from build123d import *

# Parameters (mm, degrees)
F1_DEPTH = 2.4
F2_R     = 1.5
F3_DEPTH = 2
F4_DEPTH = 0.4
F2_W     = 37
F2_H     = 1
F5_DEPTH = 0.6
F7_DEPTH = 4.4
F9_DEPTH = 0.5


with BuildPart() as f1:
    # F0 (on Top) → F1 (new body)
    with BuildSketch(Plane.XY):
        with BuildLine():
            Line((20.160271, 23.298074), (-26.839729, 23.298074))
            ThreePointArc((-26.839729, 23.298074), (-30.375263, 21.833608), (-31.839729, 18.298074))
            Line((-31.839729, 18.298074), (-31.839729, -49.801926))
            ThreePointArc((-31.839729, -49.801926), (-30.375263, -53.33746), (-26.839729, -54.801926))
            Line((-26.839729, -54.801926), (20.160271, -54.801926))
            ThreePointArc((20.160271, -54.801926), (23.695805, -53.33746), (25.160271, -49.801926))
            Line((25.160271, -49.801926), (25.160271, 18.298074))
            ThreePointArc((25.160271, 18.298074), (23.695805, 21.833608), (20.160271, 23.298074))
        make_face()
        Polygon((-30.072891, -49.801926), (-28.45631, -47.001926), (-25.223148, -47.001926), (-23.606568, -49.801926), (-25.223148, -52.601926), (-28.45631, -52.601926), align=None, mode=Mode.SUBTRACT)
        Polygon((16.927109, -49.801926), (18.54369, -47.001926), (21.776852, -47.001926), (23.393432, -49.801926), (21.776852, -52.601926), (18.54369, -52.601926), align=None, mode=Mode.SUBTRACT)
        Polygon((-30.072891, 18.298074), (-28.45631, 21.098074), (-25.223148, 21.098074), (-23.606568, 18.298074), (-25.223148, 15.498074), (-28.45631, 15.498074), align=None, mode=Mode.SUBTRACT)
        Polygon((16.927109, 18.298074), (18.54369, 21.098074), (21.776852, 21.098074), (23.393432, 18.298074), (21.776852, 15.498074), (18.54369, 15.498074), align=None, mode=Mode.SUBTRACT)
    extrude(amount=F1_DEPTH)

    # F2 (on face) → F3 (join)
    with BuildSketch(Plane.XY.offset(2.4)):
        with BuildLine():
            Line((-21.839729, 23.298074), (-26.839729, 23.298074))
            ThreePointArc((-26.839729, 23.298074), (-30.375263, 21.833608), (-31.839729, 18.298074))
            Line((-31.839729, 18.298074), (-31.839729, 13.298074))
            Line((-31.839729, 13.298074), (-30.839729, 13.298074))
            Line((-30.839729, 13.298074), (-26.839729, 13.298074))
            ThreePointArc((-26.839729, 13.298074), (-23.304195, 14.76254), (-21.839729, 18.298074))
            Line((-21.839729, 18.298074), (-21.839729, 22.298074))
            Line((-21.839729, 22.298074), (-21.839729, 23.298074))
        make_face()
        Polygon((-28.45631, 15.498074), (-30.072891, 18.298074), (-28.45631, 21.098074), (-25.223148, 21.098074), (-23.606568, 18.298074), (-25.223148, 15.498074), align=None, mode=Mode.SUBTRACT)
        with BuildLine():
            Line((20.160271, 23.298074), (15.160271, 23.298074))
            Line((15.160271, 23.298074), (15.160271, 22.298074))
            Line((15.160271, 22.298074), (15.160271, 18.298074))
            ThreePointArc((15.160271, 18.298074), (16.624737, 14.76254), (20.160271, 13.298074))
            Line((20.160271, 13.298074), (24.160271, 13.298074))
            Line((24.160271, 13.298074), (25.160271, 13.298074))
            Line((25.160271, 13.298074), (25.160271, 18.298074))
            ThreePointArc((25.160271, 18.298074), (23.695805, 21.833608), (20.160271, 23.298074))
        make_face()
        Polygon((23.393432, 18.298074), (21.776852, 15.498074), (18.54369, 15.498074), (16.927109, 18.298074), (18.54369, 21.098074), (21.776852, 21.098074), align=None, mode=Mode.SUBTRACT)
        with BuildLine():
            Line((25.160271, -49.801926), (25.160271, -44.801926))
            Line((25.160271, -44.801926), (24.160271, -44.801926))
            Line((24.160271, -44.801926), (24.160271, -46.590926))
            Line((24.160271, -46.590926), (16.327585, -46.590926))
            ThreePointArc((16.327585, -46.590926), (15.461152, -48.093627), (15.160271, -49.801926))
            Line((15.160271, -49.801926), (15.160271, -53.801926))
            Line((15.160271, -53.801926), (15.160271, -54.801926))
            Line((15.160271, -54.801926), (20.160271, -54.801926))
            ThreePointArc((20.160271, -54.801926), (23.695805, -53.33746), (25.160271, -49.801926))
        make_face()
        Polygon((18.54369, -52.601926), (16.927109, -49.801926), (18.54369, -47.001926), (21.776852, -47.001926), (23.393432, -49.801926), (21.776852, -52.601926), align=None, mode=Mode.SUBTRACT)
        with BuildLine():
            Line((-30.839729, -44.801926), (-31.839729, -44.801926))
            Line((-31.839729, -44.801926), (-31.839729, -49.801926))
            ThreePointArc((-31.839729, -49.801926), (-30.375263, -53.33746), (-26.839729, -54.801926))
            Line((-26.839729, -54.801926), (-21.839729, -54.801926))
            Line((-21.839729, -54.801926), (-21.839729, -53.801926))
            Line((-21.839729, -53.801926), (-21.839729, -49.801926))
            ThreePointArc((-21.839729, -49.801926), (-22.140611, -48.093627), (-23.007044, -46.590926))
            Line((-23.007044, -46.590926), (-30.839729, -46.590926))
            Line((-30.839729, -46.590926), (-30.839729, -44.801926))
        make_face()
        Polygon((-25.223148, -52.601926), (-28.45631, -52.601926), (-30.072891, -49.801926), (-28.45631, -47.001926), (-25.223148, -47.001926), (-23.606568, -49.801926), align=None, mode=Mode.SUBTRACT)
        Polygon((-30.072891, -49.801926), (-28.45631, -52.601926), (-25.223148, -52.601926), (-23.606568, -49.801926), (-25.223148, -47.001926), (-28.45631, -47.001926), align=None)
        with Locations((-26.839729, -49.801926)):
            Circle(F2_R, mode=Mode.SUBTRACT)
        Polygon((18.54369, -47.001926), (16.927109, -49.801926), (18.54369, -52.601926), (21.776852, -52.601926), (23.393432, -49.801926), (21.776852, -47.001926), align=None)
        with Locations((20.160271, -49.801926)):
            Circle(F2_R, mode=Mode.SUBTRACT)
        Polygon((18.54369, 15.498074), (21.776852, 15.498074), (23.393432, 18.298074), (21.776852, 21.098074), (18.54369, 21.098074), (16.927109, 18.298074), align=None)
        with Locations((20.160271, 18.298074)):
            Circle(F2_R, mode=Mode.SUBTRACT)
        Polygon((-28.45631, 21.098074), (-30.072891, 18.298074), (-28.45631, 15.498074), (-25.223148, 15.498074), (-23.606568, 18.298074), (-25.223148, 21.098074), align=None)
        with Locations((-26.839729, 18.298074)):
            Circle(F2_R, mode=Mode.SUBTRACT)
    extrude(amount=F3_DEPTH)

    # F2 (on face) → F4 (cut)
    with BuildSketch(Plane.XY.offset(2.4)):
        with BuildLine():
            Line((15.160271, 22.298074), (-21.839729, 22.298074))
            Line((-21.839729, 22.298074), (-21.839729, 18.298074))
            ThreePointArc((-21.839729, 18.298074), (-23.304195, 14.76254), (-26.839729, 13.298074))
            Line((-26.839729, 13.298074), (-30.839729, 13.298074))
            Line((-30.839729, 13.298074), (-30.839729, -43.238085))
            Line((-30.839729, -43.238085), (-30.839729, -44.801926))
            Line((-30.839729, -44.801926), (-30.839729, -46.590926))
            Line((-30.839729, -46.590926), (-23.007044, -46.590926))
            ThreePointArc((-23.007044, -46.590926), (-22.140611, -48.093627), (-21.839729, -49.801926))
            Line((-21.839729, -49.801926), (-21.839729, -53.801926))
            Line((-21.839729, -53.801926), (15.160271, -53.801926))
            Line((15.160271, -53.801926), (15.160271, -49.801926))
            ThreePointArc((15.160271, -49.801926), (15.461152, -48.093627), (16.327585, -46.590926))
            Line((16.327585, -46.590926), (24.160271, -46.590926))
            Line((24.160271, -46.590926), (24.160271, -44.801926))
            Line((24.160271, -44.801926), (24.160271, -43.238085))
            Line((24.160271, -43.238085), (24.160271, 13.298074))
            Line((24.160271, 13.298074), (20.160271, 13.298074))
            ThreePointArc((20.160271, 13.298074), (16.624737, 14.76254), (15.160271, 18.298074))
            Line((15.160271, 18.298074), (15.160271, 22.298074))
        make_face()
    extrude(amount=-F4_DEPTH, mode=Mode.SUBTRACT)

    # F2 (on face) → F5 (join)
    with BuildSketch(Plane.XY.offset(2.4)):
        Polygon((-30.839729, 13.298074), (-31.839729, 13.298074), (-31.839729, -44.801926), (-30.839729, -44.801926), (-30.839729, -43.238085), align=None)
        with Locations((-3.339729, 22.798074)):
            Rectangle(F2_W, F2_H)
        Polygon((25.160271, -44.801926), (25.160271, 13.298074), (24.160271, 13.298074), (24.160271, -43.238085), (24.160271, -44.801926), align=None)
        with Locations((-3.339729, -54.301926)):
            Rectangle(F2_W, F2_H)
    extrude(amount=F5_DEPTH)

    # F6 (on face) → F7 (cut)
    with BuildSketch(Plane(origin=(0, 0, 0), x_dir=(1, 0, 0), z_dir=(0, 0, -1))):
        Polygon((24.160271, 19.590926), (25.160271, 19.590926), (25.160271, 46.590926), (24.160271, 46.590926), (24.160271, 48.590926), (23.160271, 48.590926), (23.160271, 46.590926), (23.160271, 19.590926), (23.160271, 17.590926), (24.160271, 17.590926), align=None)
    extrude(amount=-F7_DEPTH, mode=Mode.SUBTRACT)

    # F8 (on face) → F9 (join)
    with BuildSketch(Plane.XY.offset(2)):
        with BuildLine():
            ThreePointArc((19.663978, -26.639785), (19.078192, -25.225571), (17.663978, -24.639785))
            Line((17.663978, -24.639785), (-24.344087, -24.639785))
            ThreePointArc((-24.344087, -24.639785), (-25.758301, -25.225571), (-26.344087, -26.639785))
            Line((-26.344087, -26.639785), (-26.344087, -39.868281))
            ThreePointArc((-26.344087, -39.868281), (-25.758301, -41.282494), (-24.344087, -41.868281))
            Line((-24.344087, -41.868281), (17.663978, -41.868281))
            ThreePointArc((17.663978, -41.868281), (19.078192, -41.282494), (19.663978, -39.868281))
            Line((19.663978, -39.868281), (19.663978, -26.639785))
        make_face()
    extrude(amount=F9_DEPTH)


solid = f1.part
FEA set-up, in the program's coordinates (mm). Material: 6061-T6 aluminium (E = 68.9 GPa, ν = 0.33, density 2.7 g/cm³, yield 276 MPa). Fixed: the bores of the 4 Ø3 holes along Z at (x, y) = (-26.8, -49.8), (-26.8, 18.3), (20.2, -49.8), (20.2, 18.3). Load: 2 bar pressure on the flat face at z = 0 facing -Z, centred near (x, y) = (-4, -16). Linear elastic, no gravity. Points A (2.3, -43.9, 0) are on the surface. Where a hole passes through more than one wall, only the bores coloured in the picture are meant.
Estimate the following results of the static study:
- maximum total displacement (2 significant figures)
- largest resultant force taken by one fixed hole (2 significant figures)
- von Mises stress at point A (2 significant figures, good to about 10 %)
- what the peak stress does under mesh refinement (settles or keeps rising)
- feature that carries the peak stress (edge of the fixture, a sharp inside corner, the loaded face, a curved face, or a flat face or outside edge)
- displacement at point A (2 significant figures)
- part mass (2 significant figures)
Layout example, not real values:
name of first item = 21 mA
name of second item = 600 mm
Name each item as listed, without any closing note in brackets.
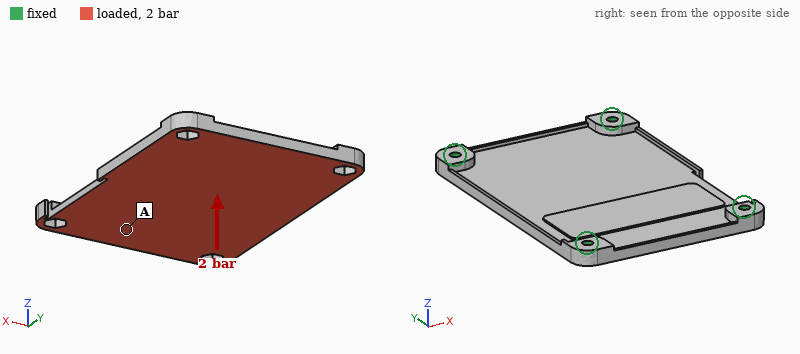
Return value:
maximum total displacement = 0.28 mm
largest resultant force taken by one fixed hole = 500 N
von Mises stress at point A = 34 MPa
what the peak stress does under mesh refinement = keeps rising
feature that carries the peak stress = edge of the fixture
displacement at point A = 0.086 mm
part mass = 26 g
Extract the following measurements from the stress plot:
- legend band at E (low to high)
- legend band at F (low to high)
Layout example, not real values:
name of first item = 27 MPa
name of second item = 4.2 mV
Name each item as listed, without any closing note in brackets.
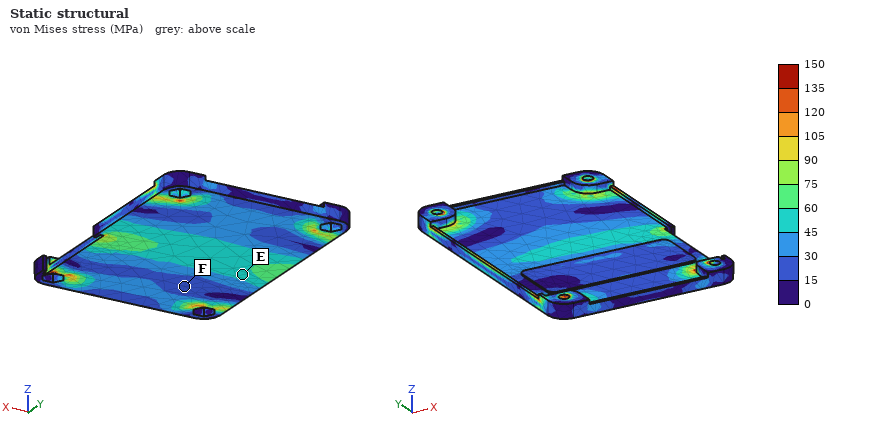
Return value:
legend band at E = 45 to 60 MPa
legend band at F = 15 to 30 MPa
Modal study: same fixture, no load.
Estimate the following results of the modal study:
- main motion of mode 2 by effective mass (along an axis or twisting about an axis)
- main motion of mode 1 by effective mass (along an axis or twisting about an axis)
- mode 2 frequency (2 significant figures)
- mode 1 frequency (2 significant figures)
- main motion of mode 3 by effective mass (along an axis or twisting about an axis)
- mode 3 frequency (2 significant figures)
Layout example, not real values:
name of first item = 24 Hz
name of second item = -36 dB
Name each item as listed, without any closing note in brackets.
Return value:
main motion of mode 2 by effective mass = twisting about Y
main motion of mode 1 by effective mass = along Z
mode 2 frequency = 3300 Hz
mode 1 frequency = 2100 Hz
main motion of mode 3 by effective mass = twisting about X
mode 3 frequency = 5100 Hz
